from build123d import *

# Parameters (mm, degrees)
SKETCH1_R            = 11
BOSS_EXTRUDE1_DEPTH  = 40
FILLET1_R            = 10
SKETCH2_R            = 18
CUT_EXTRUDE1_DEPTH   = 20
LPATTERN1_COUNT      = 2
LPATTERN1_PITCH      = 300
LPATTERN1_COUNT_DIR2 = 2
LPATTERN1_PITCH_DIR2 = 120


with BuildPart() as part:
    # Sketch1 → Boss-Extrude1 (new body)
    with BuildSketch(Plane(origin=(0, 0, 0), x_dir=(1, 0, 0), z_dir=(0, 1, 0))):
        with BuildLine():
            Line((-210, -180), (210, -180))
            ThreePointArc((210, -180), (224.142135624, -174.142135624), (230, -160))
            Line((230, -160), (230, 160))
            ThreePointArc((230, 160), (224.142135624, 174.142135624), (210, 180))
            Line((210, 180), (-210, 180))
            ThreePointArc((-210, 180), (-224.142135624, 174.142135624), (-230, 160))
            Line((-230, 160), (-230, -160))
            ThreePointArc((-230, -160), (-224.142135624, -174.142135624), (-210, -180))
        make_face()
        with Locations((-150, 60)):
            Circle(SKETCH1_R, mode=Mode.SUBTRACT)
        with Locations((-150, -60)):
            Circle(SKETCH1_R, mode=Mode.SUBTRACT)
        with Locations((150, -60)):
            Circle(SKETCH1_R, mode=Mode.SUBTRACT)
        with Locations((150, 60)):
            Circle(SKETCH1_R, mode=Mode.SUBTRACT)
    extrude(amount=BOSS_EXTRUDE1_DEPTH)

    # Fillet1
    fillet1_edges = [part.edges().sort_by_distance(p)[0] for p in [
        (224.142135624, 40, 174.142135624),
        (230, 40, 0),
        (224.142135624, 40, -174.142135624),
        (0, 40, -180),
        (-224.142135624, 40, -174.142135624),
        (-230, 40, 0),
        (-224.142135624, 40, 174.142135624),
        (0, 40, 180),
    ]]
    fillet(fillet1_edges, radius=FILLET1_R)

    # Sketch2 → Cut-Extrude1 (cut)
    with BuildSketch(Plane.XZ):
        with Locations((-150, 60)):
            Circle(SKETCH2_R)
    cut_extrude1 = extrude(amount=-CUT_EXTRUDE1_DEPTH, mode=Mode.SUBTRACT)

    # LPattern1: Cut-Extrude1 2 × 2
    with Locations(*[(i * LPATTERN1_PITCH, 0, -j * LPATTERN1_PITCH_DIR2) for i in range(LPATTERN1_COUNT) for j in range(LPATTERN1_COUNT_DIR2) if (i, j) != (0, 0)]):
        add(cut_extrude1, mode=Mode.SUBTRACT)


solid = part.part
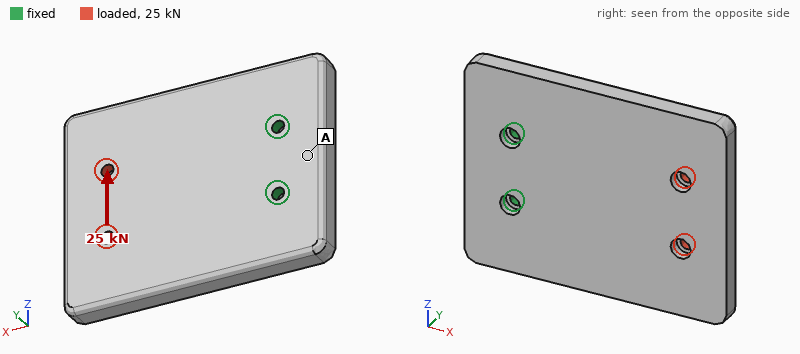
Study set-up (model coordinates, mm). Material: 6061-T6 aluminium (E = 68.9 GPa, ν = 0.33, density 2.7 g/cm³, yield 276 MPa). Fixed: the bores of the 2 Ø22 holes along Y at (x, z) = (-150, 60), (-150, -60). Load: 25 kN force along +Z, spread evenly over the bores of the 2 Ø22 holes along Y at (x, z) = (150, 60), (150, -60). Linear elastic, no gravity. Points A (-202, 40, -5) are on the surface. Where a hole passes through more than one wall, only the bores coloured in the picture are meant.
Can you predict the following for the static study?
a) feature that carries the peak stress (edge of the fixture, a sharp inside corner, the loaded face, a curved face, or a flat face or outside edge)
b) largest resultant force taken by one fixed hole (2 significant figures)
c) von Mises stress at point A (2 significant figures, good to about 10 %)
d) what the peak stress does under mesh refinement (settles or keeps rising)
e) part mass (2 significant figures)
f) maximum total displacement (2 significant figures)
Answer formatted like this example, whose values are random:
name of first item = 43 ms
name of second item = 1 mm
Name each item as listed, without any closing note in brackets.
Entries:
feature that carries the peak stress = edge of the fixture
largest resultant force taken by one fixed hole = 58 kN
von Mises stress at point A = 13 MPa
what the peak stress does under mesh refinement = keeps rising
part mass = 17 kg
maximum total displacement = 0.23 mm
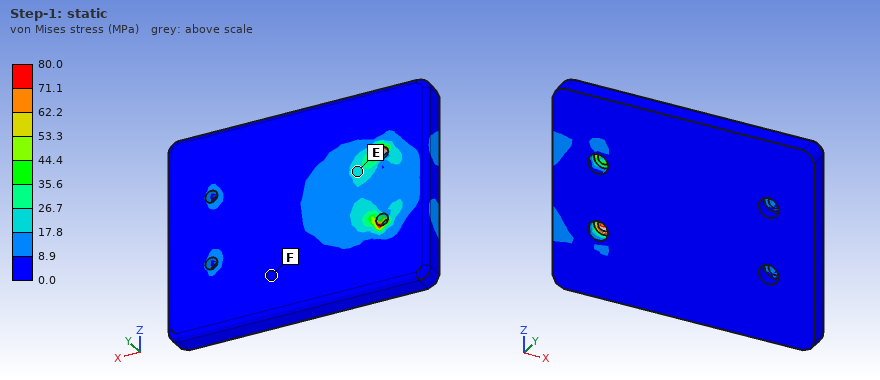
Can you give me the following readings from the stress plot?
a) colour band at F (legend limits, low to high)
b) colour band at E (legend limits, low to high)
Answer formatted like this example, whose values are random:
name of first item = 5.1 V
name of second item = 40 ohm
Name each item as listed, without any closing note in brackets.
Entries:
colour band at F = 0.0 to 8.9 MPa
colour band at E = 17.8 to 26.7 MPa
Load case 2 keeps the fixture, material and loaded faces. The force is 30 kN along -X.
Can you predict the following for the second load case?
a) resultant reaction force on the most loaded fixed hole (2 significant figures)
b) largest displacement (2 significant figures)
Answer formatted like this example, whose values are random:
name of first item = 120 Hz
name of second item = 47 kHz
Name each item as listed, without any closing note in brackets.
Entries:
resultant reaction force on the most loaded fixed hole = 15 kN
largest displacement = 0.15 mm
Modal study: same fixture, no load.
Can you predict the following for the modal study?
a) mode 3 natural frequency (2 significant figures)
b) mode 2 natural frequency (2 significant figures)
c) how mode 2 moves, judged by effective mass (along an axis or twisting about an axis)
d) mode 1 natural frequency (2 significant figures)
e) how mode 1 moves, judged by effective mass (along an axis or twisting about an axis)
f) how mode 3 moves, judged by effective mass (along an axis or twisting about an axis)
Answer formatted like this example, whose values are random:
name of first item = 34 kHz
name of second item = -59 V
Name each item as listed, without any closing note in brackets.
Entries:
mode 3 natural frequency = 690 Hz
mode 2 natural frequency = 450 Hz
how mode 2 moves, judged by effective mass = twisting about X
mode 1 natural frequency = 160 Hz
how mode 1 moves, judged by effective mass = along Y
how mode 3 moves, judged by effective mass = along Z
